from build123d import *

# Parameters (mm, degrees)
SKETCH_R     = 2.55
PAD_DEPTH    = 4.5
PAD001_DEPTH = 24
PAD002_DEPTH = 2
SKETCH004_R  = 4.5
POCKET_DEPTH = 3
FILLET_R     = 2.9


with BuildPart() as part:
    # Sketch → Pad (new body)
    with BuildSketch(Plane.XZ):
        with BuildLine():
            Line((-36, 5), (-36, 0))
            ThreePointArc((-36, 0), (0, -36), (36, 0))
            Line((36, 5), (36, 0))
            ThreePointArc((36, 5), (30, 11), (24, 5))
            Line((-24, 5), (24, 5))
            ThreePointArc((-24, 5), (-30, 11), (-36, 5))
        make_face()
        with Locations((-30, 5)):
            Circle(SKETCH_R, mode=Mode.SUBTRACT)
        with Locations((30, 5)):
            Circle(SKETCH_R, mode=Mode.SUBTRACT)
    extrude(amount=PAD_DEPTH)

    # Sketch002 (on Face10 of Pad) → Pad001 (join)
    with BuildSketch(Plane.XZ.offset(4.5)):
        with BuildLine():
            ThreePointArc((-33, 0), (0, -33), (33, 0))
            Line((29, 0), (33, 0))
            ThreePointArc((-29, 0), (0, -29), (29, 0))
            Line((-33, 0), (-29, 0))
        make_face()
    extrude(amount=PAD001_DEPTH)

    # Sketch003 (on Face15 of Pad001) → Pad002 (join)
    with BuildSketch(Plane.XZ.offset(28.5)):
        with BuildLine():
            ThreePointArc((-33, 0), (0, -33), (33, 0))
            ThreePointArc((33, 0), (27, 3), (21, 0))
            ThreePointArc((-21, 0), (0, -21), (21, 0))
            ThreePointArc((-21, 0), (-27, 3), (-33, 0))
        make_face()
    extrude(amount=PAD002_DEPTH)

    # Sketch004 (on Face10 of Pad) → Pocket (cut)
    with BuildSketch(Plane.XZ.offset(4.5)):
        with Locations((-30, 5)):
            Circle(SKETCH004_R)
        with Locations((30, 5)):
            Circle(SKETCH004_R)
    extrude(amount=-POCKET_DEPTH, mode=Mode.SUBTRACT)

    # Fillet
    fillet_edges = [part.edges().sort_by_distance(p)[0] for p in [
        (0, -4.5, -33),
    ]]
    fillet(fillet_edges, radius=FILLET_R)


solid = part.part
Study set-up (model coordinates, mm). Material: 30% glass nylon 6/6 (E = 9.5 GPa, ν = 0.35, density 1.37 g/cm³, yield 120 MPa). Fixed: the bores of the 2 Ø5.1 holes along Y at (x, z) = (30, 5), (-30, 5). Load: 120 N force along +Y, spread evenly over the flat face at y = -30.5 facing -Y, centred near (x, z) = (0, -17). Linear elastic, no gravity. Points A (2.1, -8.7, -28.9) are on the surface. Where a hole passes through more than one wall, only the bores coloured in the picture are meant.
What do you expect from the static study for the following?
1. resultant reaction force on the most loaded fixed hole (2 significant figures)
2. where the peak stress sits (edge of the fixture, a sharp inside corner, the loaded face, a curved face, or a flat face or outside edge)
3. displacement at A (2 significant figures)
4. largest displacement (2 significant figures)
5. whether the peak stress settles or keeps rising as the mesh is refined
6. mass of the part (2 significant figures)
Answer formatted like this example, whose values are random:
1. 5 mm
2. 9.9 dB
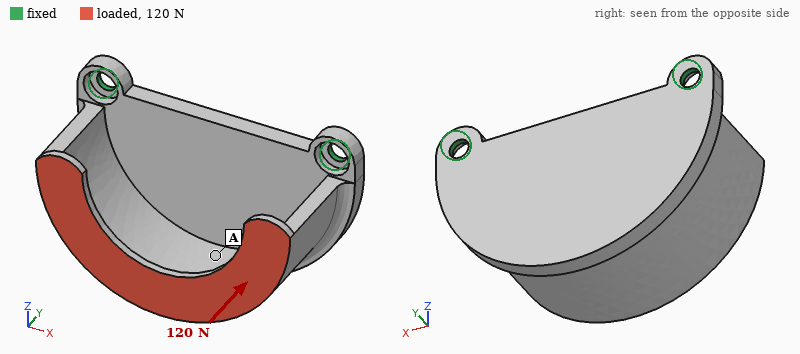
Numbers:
1. 60 N
2. edge of the fixture
3. 0.72 mm
4. 1.0 mm
5. keeps rising
6. 31 g
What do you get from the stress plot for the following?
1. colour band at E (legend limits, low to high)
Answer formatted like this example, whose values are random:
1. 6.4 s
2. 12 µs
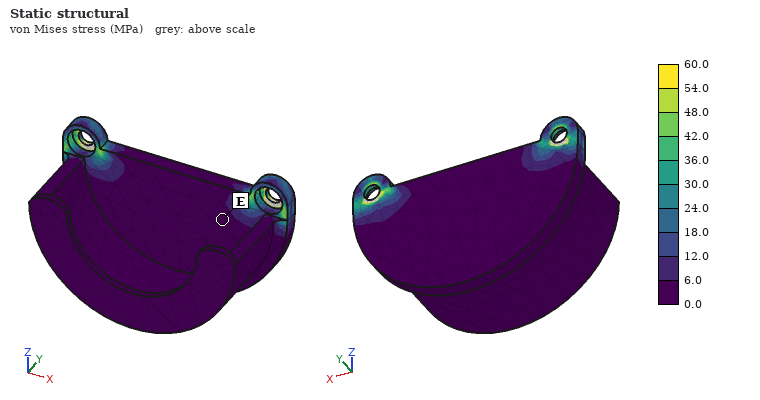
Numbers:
1. 0.0 to 6.0 MPa
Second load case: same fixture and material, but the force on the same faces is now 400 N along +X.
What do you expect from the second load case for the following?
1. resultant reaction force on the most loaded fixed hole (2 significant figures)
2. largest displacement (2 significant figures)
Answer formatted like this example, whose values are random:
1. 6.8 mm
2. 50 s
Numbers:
1. 290 N
2. 0.91 mm
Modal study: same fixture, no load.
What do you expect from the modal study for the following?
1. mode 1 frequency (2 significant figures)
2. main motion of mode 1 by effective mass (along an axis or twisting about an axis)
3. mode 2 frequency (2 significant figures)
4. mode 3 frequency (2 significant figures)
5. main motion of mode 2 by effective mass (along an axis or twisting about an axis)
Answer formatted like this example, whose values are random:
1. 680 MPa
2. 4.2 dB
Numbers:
1. 360 Hz
2. along Y
3. 1300 Hz
4. 3300 Hz
5. along X
